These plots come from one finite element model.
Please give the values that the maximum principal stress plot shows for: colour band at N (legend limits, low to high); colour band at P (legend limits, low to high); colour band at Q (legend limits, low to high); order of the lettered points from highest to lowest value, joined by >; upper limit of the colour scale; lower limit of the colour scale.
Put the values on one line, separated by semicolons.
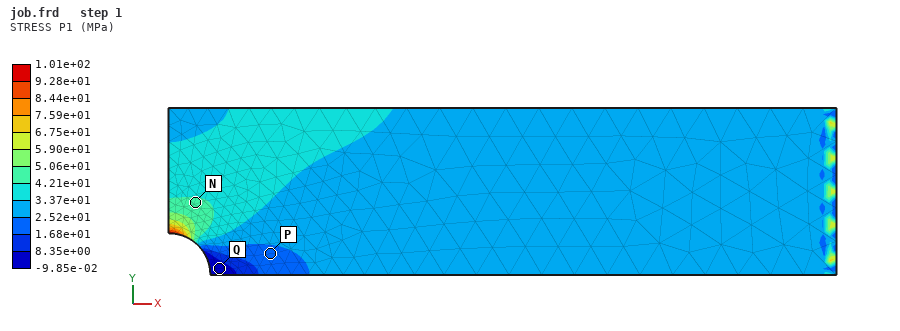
4.21e+01 to 5.06e+01 MPa; 1.68e+01 to 2.52e+01 MPa; -9.85e-02 to 8.35e+00 MPa; N > P > Q; 1.01e+02 MPa; -9.85e-02 MPa
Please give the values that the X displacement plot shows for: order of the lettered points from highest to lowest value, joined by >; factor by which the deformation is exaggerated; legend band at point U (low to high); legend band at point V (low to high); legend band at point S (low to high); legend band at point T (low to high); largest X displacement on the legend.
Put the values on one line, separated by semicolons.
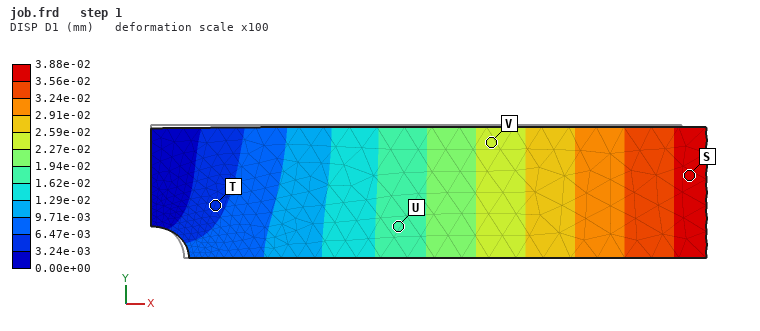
S > V > U > T; 100; 1.62e-02 to 1.94e-02 mm; 2.27e-02 to 2.59e-02 mm; 3.56e-02 to 3.88e-02 mm; 3.24e-03 to 6.47e-03 mm; 3.88e-02 mm
